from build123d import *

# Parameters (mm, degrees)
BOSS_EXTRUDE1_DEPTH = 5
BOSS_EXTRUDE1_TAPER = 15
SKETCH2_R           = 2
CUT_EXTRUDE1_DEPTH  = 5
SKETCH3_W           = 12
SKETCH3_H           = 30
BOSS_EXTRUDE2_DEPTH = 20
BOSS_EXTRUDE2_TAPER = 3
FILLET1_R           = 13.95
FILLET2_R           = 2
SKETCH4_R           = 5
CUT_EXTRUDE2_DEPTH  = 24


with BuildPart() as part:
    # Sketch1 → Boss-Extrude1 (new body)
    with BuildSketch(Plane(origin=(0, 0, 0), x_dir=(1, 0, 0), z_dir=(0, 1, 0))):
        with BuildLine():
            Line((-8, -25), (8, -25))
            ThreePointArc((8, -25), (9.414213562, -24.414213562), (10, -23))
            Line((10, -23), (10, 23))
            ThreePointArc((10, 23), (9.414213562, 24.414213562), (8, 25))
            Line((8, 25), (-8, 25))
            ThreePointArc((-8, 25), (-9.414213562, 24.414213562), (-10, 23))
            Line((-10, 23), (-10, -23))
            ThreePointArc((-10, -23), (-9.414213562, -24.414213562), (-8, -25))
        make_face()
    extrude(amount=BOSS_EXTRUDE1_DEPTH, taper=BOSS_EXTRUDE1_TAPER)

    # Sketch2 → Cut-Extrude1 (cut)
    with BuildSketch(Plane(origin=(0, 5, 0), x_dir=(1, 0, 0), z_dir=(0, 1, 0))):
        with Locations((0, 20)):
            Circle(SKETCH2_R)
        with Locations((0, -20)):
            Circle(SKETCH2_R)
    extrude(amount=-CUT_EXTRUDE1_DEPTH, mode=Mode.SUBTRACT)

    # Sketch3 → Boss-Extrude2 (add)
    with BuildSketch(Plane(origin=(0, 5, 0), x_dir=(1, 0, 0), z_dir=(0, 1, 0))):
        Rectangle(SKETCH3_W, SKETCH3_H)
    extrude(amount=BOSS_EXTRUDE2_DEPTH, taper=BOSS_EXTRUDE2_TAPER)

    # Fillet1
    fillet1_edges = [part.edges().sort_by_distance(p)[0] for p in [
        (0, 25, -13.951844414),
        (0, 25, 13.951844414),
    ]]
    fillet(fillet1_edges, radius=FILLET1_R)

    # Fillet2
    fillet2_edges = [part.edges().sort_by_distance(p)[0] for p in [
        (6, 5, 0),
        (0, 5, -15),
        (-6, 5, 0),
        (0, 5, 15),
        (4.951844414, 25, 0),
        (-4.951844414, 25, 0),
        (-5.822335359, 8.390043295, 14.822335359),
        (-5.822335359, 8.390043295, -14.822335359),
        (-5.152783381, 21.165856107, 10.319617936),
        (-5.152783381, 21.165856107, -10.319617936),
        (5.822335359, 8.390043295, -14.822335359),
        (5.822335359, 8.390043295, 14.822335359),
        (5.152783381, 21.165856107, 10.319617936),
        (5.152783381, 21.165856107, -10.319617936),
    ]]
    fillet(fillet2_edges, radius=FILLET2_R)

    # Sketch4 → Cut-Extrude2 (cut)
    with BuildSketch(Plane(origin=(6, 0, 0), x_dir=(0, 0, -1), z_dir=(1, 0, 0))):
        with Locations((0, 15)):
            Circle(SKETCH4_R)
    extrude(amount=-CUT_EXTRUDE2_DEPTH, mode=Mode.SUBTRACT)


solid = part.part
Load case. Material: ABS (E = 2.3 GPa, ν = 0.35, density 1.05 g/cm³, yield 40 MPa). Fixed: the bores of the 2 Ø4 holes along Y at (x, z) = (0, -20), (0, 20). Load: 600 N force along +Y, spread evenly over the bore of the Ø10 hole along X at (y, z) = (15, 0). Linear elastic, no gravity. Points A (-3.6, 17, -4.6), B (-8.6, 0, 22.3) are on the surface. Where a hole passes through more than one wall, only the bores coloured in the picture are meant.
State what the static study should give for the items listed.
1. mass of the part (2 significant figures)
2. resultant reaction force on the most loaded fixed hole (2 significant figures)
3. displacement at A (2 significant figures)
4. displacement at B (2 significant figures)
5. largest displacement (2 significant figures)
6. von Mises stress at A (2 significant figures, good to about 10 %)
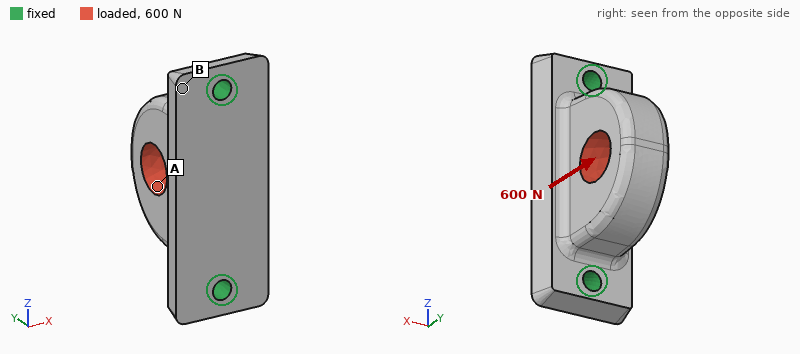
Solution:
9.6 g
340 N
90 µm
20 µm
99 µm
4.2 MPa
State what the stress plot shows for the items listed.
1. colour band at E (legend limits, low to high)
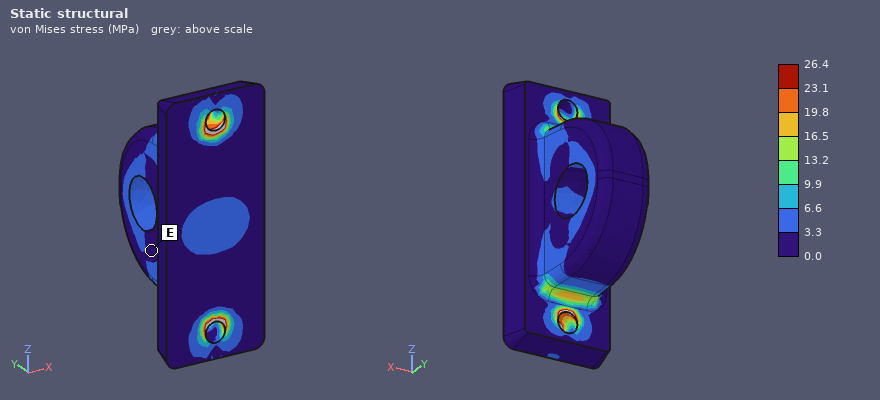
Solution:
0.0 to 3.3 MPa
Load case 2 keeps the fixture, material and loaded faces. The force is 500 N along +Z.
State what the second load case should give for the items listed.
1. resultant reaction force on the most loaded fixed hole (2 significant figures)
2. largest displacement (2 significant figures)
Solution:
310 N
90 µm
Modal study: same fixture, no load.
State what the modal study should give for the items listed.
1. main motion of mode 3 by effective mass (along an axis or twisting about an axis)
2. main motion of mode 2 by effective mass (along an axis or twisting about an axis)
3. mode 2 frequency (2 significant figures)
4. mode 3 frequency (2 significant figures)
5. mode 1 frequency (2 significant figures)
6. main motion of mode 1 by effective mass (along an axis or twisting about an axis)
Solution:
along Z
along Y
4800 Hz
6300 Hz
2200 Hz
along X
